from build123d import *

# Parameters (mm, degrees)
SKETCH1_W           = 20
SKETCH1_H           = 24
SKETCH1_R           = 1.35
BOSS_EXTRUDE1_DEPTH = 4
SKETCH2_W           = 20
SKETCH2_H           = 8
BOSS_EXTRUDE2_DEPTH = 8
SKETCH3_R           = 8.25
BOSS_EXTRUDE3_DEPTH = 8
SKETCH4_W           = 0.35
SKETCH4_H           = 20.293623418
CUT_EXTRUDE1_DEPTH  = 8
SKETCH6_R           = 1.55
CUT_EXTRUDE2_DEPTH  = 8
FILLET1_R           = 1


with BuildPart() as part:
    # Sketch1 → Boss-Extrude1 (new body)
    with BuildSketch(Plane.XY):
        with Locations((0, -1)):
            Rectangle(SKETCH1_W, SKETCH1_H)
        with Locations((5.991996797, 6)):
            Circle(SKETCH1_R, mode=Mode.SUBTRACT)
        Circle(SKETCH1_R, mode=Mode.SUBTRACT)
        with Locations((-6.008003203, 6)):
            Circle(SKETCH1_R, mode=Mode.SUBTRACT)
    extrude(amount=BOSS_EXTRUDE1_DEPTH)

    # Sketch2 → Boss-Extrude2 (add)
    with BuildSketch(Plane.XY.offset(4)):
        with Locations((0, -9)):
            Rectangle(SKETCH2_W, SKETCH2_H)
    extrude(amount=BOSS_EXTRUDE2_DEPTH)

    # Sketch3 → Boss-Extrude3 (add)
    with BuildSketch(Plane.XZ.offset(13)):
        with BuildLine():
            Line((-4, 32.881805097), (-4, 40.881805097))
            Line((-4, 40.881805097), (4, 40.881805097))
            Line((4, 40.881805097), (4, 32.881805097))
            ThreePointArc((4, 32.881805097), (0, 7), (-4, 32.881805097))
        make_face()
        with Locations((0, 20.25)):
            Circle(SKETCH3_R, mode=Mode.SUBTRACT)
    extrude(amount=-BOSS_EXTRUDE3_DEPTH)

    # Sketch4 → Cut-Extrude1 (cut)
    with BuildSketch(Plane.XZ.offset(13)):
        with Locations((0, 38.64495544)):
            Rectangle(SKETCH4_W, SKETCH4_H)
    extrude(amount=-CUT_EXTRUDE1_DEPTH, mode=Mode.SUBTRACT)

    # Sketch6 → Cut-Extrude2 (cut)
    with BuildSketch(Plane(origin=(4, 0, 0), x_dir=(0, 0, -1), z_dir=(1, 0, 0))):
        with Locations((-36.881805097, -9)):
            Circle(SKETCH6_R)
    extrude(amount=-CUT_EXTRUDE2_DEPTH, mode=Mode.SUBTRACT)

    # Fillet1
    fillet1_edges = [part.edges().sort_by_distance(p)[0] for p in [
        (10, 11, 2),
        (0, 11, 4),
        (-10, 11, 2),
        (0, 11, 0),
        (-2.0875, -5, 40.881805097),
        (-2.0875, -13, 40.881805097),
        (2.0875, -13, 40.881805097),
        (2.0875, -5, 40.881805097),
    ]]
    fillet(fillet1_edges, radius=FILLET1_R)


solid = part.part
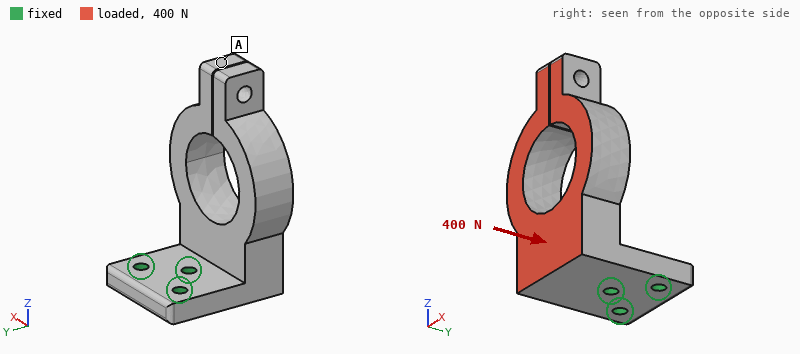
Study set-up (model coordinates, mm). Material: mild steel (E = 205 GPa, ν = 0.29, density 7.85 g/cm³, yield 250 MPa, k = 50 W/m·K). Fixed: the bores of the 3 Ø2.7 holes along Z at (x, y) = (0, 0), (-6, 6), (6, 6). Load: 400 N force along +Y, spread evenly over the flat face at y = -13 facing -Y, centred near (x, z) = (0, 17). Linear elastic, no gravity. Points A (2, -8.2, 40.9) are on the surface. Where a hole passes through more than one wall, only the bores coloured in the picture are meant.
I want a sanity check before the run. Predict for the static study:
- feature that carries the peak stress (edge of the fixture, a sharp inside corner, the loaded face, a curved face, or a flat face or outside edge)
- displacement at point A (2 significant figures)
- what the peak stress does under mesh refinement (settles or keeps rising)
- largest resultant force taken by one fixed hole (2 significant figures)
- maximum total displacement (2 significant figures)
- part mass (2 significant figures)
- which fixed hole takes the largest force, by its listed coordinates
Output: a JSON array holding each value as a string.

["edge of the fixture", "0.098 mm", "keeps rising", "490 N", "0.10 mm", "44 g", "(0, 0)"]
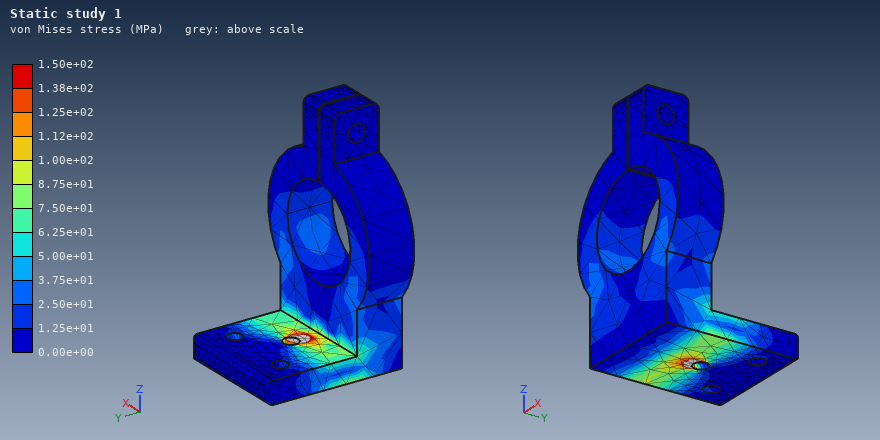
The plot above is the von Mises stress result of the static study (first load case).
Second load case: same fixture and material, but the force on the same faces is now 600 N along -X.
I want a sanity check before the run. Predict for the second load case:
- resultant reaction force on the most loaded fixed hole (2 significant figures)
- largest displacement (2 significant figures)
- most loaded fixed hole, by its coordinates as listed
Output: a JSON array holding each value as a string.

["710 N", "92 µm", "(0, 0)"]
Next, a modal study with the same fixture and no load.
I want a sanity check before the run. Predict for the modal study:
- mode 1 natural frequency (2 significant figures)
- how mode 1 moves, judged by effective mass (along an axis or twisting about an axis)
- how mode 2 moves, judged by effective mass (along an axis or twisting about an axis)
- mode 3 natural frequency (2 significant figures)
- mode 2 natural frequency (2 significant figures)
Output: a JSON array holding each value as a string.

["2100 Hz", "along Y", "along X", "4200 Hz", "2800 Hz"]
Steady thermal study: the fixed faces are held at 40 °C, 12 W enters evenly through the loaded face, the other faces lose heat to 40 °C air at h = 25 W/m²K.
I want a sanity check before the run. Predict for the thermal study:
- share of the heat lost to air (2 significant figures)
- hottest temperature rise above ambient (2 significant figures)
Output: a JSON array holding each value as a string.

["17 %", "50 K"]
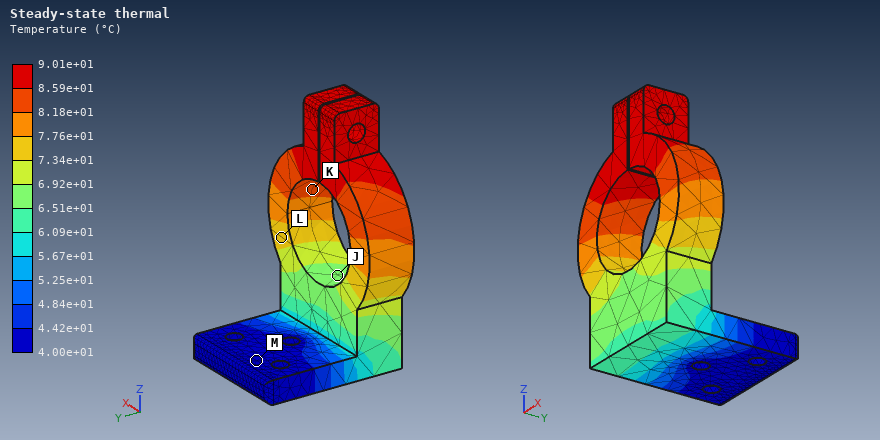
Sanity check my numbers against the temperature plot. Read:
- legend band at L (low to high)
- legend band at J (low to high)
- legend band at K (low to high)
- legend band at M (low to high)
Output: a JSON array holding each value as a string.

["7.34e+01 to 7.76e+01 °C", "6.51e+01 to 6.92e+01 °C", "8.18e+01 to 8.59e+01 °C", "4.00e+01 to 4.42e+01 °C"]
